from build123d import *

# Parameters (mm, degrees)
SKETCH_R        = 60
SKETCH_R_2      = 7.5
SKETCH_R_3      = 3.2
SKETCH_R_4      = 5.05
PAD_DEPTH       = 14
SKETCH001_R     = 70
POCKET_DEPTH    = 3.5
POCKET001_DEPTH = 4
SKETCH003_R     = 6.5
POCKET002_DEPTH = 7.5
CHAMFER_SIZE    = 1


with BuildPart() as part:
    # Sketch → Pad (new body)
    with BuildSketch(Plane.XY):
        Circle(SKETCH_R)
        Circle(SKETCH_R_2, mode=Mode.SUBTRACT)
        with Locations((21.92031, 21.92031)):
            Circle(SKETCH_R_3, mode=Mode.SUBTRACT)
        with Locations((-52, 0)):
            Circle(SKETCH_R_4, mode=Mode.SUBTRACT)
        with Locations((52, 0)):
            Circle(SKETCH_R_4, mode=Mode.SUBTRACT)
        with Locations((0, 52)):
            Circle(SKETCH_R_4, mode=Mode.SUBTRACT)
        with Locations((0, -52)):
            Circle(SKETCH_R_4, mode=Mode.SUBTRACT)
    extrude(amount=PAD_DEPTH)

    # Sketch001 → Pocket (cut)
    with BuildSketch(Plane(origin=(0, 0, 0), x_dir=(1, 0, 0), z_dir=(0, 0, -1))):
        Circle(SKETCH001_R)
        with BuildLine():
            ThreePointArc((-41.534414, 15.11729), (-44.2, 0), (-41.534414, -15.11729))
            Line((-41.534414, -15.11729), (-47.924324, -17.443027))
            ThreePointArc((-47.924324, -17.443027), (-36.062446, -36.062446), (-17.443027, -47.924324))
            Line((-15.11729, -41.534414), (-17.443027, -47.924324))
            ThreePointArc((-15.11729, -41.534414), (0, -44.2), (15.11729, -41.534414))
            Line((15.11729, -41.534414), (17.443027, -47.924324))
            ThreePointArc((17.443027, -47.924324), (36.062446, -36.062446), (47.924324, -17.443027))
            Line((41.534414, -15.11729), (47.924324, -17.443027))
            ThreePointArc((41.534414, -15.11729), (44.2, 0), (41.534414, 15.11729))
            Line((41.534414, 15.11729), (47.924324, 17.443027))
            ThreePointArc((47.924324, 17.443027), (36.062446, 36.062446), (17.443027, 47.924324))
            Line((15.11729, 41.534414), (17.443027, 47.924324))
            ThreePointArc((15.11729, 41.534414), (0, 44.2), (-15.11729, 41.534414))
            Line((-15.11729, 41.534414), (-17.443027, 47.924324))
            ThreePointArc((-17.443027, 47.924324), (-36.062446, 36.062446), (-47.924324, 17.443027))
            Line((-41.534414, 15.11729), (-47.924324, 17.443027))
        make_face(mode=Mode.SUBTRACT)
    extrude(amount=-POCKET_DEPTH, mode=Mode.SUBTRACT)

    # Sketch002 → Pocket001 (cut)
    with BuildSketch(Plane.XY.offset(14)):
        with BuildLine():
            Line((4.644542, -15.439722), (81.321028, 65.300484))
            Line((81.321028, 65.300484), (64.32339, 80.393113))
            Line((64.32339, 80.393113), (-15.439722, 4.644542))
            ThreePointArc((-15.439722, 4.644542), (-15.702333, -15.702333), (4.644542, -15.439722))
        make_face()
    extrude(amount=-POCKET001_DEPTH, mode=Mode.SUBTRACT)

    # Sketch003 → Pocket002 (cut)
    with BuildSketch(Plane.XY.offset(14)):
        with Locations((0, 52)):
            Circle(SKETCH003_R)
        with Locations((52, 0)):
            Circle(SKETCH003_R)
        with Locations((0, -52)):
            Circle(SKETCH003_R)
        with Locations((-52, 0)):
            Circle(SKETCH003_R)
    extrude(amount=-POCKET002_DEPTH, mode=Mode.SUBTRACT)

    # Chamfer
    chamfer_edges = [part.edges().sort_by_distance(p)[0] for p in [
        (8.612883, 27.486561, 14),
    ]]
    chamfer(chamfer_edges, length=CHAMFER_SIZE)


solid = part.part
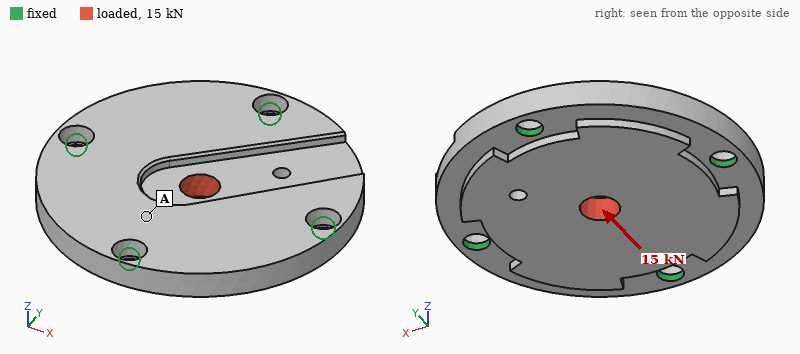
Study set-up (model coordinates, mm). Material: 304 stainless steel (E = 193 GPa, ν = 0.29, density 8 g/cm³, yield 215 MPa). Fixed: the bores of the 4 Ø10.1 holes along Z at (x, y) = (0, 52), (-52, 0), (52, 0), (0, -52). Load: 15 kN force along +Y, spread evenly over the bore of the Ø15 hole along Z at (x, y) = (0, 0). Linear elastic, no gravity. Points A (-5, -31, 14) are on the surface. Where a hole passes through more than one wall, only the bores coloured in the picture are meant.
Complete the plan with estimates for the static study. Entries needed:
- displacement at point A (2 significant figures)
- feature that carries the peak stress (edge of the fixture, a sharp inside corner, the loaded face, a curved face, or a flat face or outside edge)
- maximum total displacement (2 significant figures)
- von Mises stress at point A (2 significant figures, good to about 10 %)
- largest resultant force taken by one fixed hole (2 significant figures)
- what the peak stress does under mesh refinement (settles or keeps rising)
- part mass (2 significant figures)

2.8 µm
edge of the fixture
6.2 µm
11 MPa
4.6 kN
keeps rising
1.0 kg
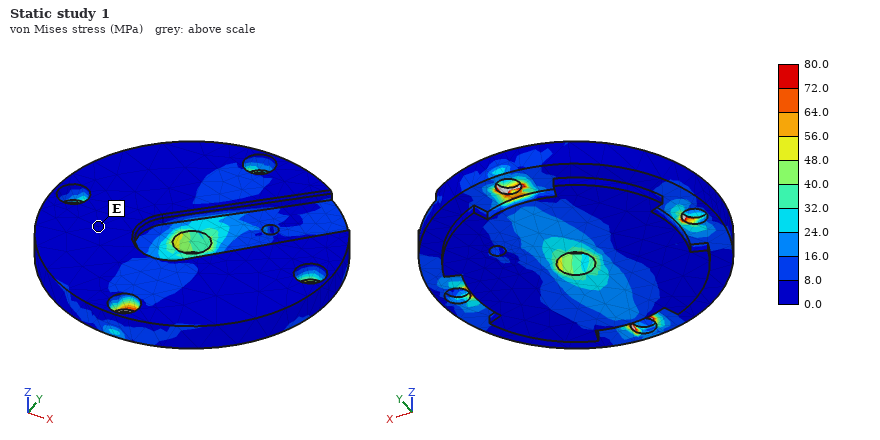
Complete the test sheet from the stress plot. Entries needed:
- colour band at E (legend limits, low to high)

0.0 to 8.0 MPa
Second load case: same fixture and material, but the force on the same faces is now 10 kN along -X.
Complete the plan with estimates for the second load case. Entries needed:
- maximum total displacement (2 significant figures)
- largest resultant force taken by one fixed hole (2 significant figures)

4.1 µm
3.1 kN
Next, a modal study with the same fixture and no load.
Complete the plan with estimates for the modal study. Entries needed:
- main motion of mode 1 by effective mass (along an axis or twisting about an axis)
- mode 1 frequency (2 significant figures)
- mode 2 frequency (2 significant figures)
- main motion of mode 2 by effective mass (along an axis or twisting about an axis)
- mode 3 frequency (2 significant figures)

along Z
5200 Hz
6000 Hz
along Z
6800 Hz
